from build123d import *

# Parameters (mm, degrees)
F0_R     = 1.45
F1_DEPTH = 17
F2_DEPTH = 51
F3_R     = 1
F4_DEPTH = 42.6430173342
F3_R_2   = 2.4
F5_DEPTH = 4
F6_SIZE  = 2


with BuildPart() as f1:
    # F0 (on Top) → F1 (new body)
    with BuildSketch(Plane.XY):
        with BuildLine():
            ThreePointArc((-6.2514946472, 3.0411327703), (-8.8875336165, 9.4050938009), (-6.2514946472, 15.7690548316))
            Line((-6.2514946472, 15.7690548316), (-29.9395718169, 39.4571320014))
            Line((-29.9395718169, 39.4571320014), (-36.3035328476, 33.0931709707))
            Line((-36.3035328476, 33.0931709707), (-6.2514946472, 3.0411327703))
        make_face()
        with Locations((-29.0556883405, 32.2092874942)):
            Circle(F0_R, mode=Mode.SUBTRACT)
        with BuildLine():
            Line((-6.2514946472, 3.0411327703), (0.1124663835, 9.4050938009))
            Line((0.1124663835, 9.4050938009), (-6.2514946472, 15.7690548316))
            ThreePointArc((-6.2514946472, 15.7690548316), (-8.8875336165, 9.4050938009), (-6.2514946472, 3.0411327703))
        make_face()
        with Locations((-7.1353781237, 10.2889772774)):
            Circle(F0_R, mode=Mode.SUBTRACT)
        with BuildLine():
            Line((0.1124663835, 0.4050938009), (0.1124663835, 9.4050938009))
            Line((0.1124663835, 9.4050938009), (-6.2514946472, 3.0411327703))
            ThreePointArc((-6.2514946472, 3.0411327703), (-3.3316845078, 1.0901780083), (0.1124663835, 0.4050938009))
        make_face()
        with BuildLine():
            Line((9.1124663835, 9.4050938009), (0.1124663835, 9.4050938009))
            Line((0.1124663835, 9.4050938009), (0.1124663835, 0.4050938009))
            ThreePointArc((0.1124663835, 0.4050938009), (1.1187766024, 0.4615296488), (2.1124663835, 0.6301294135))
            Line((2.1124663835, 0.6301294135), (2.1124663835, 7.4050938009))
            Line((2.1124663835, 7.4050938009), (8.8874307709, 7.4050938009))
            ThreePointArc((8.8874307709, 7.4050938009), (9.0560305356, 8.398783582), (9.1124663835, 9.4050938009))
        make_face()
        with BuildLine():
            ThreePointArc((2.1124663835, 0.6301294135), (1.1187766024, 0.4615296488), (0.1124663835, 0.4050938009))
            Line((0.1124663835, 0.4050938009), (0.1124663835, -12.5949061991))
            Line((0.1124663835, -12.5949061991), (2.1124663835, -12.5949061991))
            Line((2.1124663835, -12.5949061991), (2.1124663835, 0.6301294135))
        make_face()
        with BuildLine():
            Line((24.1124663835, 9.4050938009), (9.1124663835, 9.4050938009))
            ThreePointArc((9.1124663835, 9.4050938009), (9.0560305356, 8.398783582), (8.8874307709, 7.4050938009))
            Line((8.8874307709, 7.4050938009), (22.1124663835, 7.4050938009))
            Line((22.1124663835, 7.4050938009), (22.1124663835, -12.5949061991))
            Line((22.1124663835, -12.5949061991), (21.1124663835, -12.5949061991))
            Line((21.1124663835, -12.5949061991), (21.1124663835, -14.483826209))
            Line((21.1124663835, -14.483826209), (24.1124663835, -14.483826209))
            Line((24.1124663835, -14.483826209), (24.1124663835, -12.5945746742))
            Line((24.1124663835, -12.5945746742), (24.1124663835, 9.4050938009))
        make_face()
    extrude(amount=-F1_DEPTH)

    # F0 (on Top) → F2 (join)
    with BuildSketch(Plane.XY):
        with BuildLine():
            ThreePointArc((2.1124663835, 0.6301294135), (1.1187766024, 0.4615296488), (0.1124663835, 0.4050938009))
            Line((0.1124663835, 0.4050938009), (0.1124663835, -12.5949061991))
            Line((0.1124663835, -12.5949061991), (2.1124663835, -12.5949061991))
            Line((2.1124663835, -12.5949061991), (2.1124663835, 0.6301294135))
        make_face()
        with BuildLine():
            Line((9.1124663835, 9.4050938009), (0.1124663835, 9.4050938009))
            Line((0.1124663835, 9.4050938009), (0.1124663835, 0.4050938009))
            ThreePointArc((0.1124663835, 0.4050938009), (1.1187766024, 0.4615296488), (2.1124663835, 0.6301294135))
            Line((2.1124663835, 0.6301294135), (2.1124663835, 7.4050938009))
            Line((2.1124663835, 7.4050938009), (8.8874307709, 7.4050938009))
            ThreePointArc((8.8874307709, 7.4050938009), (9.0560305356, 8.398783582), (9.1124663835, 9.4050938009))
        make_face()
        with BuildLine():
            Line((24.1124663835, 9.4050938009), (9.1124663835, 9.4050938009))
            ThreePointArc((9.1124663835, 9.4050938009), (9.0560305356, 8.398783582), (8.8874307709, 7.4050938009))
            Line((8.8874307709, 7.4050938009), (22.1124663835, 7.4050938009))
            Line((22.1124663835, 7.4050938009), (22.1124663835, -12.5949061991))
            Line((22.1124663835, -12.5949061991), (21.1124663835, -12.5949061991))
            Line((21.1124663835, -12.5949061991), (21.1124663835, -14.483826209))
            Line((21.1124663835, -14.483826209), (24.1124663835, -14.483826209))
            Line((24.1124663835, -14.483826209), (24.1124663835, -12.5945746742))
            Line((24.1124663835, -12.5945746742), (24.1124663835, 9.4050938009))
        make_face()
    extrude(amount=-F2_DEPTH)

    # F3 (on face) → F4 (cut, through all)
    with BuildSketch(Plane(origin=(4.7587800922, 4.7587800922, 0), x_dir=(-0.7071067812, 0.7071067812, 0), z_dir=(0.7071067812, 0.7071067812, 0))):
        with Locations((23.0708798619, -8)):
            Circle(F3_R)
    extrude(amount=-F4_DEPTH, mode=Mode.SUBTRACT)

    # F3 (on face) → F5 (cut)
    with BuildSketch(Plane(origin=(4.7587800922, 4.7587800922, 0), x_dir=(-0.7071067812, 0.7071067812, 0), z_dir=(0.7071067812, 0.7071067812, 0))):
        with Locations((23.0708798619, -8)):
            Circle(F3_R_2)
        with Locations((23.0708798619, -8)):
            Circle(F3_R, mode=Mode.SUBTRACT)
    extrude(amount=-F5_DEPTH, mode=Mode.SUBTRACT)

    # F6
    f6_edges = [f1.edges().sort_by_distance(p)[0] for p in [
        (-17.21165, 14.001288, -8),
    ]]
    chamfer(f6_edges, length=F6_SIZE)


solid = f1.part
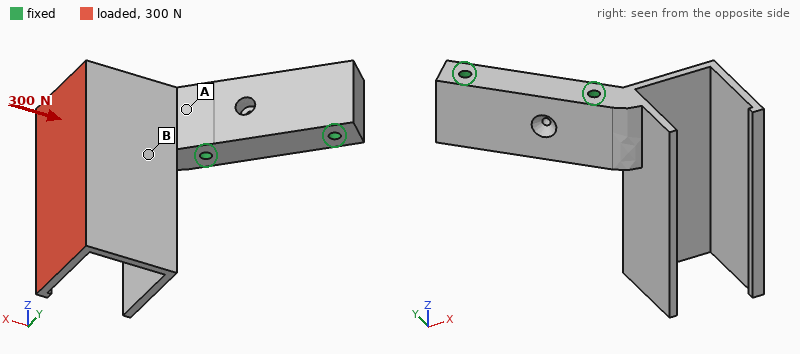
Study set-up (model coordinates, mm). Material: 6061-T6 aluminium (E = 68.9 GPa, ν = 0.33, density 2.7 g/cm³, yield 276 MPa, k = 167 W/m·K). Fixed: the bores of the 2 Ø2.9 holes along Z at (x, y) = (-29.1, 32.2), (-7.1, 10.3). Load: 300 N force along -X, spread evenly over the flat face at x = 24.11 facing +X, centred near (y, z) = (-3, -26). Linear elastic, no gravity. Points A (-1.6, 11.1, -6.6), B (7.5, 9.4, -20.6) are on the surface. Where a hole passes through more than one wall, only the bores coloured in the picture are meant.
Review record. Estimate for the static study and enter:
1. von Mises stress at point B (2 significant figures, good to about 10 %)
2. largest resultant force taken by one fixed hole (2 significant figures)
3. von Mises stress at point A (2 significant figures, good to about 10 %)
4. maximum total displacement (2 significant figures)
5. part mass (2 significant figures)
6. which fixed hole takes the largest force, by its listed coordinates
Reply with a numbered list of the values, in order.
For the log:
1. 87 MPa
2. 330 N
3. 19 MPa
4. 1.1 mm
5. 37 g
6. (-7.1, 10.3)
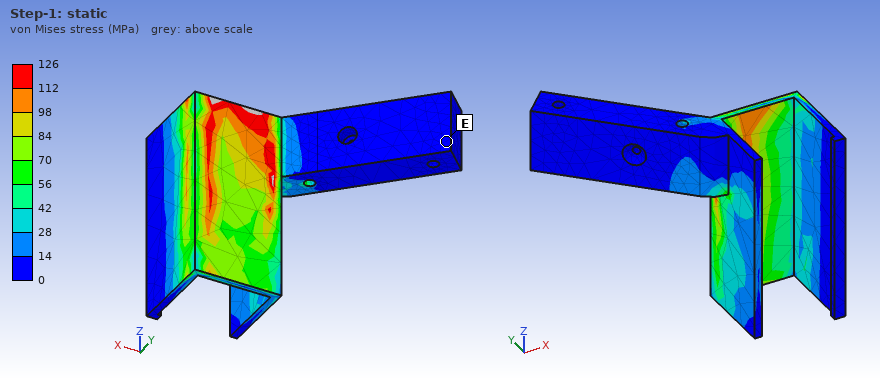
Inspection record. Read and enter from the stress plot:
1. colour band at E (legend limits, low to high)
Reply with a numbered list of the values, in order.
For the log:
1. 0 to 14 MPa
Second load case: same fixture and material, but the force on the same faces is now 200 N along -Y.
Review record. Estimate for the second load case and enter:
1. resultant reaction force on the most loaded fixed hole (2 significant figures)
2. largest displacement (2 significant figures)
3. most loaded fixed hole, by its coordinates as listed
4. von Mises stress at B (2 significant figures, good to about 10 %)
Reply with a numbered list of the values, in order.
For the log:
1. 270 N
2. 1.1 mm
3. (-7.1, 10.3)
4. 110 MPa
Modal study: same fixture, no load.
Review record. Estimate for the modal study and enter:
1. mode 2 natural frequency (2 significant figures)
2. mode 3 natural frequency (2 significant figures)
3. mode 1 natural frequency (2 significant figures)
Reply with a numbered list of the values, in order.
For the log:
1. 1600 Hz
2. 2600 Hz
3. 850 Hz
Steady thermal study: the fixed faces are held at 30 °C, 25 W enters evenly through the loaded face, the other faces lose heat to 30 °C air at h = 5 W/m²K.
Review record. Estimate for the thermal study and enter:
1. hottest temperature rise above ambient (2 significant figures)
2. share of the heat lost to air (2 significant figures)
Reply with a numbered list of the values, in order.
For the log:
1. 71 K
2. 4.7 %
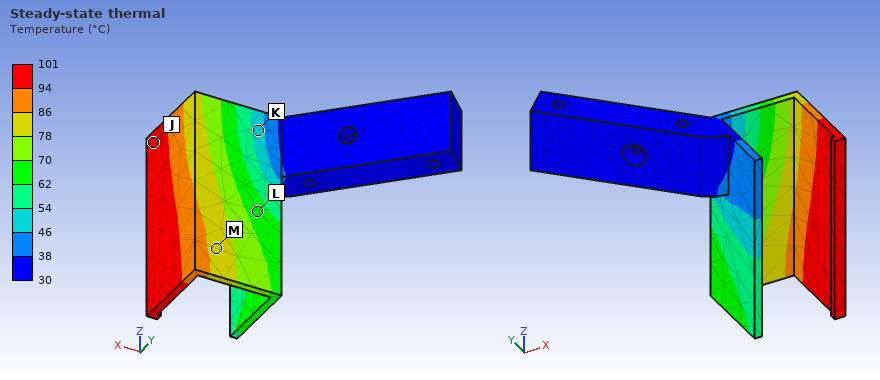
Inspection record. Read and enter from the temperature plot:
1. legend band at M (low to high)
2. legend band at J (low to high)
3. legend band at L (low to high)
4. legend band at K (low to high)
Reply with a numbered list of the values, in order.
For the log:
1. 78 to 86 °C
2. 94 to 101 °C
3. 62 to 70 °C
4. 46 to 54 °C
